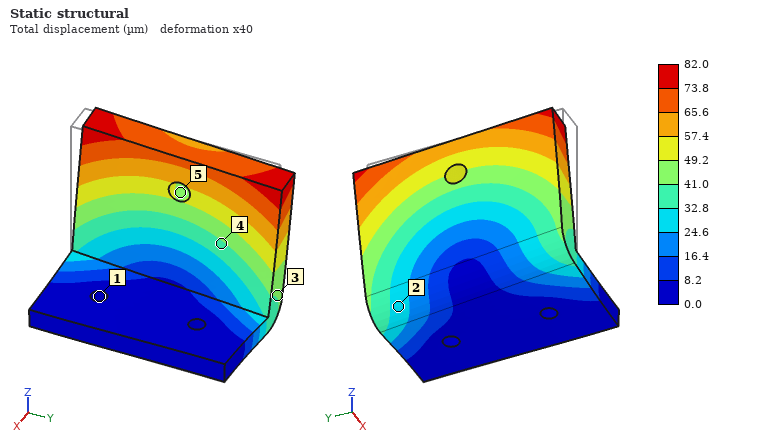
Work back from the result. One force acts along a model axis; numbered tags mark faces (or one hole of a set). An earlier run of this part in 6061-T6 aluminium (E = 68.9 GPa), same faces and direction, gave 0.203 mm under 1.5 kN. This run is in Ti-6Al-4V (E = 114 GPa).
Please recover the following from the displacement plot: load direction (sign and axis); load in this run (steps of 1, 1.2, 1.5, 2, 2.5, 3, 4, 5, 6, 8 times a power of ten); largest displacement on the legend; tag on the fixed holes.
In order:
+Y
1 kN
82.0 µm
1
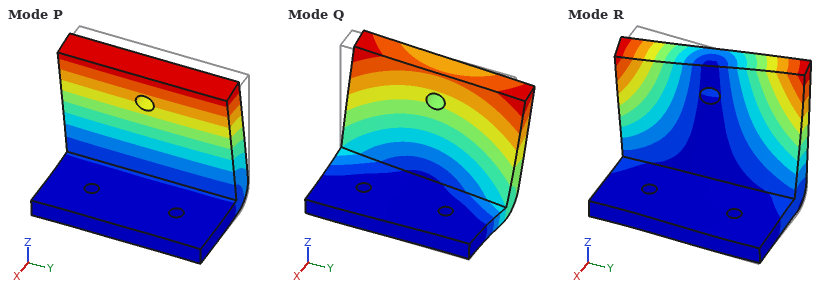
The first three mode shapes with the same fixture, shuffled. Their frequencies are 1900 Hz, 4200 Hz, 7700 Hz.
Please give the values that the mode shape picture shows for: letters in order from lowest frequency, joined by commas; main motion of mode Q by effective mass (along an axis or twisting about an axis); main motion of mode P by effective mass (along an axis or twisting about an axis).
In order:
P, Q, R
along Y
along X
